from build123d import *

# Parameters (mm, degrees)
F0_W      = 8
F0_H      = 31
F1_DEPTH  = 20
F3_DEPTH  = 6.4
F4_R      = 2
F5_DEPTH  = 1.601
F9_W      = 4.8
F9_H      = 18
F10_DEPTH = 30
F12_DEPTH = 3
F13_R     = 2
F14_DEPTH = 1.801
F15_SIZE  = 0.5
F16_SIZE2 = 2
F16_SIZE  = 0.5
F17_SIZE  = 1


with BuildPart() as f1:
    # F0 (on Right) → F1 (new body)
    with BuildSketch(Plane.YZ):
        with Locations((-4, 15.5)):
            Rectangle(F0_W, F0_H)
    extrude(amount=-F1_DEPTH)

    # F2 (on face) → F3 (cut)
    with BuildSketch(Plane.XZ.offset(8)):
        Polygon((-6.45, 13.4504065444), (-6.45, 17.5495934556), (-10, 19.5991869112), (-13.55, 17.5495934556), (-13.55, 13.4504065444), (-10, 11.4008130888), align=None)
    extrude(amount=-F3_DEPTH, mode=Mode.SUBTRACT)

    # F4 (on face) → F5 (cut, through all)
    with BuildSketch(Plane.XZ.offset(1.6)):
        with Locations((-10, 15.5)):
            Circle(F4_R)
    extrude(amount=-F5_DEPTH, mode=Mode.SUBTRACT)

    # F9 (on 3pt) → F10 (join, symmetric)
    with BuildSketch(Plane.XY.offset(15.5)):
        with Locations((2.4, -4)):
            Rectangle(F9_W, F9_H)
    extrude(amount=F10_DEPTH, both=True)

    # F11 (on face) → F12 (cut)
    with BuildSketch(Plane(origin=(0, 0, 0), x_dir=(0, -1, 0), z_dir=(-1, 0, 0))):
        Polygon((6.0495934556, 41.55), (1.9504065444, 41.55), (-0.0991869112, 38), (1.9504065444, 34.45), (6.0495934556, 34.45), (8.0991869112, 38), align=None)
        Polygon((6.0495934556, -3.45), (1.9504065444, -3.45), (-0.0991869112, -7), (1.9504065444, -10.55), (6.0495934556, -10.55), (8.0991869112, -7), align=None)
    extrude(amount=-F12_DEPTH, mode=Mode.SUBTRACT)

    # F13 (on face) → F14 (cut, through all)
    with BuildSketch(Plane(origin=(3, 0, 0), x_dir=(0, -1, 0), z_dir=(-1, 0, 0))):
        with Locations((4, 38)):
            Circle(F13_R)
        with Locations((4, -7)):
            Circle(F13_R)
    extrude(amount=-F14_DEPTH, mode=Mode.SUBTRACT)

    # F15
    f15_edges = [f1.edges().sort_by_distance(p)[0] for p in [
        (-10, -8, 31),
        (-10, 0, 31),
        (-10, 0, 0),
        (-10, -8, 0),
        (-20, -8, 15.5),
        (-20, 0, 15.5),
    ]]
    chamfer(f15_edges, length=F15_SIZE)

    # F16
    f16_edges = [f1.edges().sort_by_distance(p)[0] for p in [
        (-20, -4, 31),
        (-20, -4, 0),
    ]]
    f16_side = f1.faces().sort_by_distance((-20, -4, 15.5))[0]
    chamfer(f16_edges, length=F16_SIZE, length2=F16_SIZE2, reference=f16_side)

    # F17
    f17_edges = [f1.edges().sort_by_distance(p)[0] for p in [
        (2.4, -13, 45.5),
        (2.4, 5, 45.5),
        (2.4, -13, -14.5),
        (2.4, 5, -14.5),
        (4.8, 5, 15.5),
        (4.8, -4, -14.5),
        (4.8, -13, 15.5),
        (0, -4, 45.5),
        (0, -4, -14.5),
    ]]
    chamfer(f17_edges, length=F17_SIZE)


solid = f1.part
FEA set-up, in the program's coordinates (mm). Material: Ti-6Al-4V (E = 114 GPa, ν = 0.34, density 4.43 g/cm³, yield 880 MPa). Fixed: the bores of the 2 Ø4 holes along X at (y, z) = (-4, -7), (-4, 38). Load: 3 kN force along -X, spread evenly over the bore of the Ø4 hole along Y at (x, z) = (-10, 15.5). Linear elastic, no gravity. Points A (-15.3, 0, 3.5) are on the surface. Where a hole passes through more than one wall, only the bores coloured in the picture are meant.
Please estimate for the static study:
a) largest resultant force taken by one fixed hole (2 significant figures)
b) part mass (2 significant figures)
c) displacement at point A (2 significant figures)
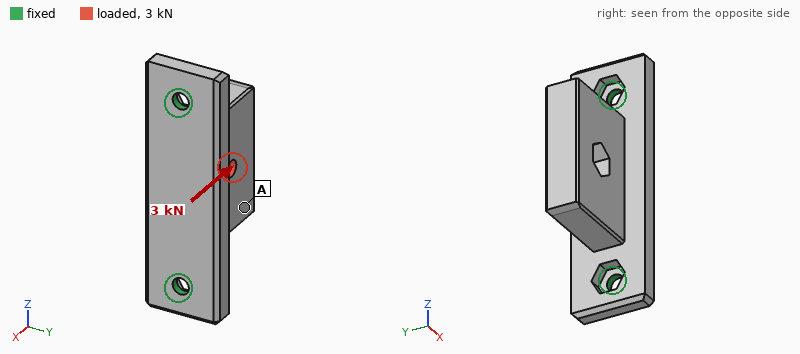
2.1 kN
42 g
0.10 mm
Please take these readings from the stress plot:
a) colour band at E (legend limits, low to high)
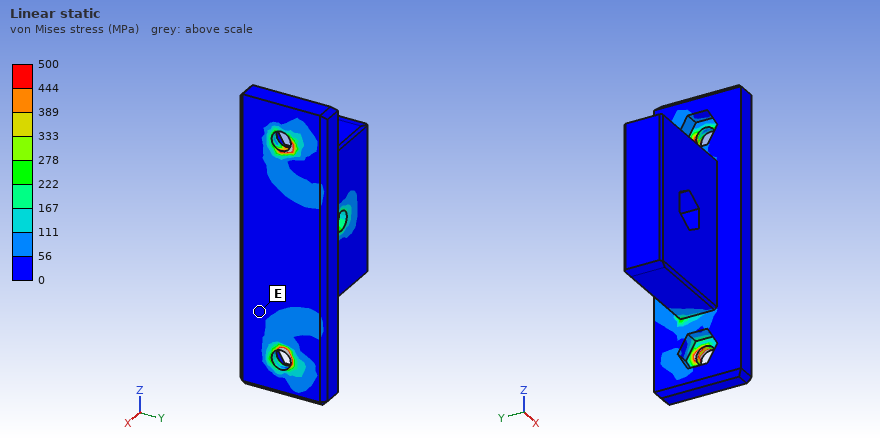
0 to 56 MPa
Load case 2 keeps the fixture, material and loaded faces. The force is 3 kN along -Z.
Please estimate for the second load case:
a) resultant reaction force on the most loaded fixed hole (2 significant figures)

1.8 kN
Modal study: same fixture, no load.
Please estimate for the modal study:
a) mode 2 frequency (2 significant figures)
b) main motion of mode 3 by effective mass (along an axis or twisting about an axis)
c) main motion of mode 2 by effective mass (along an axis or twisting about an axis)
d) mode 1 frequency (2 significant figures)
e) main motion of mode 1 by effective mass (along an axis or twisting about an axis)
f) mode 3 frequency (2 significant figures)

9700 Hz
along Z
along X
3100 Hz
along Y
13 kHz
